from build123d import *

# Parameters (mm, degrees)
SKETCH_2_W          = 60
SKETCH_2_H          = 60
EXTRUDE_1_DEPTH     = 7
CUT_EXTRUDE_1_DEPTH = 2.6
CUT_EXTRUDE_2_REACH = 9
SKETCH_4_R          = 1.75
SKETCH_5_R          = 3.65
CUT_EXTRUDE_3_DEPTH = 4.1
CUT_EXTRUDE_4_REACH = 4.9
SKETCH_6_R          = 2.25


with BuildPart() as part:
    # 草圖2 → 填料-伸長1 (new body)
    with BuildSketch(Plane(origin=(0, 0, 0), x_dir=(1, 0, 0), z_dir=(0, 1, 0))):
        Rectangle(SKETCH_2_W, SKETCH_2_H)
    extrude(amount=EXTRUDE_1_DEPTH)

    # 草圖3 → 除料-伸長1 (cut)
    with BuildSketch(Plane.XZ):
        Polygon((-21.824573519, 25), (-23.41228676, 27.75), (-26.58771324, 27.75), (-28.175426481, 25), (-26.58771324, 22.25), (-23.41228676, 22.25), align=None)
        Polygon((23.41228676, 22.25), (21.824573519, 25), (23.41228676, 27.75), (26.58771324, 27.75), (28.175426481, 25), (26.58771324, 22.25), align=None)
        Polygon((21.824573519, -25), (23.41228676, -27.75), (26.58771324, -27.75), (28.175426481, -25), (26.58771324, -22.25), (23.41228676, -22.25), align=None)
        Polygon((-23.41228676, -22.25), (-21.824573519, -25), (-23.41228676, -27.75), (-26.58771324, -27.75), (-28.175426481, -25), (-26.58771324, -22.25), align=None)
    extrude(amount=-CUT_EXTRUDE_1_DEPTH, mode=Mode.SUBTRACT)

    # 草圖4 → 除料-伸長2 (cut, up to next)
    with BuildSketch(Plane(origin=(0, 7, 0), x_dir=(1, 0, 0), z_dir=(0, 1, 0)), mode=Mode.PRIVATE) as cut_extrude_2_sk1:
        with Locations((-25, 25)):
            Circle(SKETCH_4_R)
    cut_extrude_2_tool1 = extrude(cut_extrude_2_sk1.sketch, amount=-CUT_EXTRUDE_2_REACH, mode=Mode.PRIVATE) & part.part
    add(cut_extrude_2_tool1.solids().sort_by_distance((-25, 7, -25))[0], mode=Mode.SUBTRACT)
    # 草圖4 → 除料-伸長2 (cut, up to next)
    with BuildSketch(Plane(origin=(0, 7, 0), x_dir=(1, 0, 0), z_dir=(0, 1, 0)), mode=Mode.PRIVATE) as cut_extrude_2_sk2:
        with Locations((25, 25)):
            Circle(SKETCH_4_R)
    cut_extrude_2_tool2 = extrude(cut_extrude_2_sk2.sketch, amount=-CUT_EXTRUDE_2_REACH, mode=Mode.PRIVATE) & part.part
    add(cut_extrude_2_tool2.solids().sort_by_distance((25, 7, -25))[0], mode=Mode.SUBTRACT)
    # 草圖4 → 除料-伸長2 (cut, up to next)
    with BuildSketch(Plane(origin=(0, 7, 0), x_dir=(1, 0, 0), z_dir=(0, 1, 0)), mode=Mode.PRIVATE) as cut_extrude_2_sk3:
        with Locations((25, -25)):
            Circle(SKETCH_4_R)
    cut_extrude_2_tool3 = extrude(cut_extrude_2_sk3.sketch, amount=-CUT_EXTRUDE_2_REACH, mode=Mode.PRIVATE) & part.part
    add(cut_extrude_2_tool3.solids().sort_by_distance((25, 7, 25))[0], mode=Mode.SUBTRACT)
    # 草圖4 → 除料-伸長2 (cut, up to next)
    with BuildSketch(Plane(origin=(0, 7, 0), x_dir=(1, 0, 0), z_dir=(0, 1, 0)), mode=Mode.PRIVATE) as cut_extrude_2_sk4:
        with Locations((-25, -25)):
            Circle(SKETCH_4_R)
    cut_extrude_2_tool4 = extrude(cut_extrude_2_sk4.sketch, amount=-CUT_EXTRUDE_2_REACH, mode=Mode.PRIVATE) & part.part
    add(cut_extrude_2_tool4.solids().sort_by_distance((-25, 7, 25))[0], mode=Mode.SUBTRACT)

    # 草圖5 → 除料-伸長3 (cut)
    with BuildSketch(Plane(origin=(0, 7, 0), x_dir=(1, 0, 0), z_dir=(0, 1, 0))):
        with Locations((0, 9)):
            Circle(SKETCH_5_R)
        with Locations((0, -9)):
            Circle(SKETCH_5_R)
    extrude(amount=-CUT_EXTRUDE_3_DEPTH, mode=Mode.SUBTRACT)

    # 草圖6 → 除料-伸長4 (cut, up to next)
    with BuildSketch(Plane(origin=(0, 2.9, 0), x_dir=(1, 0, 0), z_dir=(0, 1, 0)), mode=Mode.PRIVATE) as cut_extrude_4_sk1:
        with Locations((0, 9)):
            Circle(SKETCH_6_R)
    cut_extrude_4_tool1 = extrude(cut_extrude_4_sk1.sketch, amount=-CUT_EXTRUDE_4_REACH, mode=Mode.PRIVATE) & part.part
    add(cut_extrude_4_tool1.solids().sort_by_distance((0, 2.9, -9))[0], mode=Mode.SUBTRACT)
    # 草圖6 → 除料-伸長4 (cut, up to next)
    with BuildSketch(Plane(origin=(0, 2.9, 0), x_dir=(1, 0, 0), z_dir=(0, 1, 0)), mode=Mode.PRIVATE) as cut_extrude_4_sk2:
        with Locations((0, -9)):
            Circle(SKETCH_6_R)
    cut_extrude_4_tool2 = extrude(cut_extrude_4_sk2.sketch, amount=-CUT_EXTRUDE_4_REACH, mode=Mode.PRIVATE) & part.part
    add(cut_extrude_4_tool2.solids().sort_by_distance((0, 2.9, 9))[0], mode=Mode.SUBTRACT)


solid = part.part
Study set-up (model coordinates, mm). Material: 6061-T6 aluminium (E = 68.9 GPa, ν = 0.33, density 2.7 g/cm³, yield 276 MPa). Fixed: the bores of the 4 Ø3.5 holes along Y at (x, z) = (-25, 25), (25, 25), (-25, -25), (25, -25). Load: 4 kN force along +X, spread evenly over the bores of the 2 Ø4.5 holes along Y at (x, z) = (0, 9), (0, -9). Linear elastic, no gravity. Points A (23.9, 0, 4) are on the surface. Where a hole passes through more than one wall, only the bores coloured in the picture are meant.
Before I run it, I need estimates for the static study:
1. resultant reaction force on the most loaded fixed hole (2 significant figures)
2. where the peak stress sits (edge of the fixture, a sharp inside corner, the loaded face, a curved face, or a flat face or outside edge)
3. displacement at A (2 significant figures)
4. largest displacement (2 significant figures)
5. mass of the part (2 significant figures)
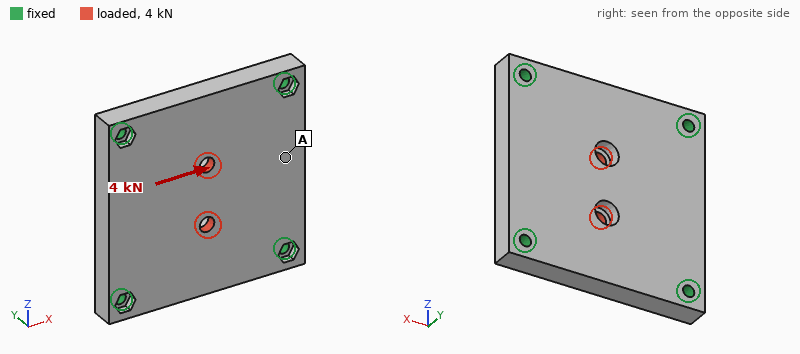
1.1 kN
a sharp inside corner
5.3 µm
9.0 µm
66 g
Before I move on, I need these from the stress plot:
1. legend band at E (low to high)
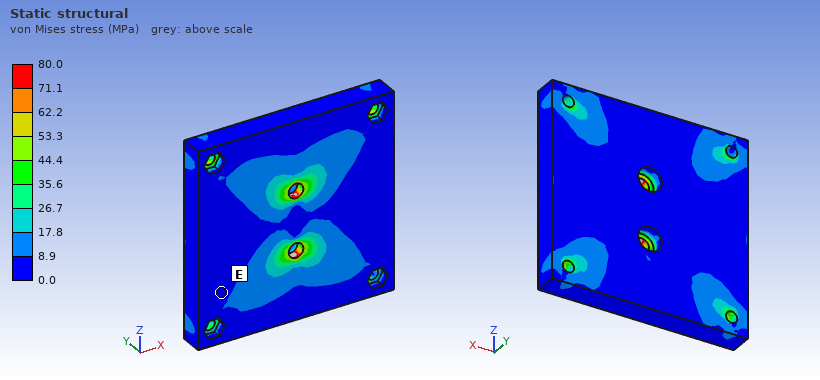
0.0 to 8.9 MPa
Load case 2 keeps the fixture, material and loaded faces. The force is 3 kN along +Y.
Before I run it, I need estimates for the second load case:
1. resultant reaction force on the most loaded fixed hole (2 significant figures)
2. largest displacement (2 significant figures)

1.1 kN
73 µm
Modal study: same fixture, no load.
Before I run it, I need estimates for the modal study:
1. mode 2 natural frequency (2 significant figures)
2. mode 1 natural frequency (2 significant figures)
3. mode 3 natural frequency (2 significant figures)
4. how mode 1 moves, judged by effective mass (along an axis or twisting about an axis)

12 kHz
7400 Hz
12 kHz
along Y
